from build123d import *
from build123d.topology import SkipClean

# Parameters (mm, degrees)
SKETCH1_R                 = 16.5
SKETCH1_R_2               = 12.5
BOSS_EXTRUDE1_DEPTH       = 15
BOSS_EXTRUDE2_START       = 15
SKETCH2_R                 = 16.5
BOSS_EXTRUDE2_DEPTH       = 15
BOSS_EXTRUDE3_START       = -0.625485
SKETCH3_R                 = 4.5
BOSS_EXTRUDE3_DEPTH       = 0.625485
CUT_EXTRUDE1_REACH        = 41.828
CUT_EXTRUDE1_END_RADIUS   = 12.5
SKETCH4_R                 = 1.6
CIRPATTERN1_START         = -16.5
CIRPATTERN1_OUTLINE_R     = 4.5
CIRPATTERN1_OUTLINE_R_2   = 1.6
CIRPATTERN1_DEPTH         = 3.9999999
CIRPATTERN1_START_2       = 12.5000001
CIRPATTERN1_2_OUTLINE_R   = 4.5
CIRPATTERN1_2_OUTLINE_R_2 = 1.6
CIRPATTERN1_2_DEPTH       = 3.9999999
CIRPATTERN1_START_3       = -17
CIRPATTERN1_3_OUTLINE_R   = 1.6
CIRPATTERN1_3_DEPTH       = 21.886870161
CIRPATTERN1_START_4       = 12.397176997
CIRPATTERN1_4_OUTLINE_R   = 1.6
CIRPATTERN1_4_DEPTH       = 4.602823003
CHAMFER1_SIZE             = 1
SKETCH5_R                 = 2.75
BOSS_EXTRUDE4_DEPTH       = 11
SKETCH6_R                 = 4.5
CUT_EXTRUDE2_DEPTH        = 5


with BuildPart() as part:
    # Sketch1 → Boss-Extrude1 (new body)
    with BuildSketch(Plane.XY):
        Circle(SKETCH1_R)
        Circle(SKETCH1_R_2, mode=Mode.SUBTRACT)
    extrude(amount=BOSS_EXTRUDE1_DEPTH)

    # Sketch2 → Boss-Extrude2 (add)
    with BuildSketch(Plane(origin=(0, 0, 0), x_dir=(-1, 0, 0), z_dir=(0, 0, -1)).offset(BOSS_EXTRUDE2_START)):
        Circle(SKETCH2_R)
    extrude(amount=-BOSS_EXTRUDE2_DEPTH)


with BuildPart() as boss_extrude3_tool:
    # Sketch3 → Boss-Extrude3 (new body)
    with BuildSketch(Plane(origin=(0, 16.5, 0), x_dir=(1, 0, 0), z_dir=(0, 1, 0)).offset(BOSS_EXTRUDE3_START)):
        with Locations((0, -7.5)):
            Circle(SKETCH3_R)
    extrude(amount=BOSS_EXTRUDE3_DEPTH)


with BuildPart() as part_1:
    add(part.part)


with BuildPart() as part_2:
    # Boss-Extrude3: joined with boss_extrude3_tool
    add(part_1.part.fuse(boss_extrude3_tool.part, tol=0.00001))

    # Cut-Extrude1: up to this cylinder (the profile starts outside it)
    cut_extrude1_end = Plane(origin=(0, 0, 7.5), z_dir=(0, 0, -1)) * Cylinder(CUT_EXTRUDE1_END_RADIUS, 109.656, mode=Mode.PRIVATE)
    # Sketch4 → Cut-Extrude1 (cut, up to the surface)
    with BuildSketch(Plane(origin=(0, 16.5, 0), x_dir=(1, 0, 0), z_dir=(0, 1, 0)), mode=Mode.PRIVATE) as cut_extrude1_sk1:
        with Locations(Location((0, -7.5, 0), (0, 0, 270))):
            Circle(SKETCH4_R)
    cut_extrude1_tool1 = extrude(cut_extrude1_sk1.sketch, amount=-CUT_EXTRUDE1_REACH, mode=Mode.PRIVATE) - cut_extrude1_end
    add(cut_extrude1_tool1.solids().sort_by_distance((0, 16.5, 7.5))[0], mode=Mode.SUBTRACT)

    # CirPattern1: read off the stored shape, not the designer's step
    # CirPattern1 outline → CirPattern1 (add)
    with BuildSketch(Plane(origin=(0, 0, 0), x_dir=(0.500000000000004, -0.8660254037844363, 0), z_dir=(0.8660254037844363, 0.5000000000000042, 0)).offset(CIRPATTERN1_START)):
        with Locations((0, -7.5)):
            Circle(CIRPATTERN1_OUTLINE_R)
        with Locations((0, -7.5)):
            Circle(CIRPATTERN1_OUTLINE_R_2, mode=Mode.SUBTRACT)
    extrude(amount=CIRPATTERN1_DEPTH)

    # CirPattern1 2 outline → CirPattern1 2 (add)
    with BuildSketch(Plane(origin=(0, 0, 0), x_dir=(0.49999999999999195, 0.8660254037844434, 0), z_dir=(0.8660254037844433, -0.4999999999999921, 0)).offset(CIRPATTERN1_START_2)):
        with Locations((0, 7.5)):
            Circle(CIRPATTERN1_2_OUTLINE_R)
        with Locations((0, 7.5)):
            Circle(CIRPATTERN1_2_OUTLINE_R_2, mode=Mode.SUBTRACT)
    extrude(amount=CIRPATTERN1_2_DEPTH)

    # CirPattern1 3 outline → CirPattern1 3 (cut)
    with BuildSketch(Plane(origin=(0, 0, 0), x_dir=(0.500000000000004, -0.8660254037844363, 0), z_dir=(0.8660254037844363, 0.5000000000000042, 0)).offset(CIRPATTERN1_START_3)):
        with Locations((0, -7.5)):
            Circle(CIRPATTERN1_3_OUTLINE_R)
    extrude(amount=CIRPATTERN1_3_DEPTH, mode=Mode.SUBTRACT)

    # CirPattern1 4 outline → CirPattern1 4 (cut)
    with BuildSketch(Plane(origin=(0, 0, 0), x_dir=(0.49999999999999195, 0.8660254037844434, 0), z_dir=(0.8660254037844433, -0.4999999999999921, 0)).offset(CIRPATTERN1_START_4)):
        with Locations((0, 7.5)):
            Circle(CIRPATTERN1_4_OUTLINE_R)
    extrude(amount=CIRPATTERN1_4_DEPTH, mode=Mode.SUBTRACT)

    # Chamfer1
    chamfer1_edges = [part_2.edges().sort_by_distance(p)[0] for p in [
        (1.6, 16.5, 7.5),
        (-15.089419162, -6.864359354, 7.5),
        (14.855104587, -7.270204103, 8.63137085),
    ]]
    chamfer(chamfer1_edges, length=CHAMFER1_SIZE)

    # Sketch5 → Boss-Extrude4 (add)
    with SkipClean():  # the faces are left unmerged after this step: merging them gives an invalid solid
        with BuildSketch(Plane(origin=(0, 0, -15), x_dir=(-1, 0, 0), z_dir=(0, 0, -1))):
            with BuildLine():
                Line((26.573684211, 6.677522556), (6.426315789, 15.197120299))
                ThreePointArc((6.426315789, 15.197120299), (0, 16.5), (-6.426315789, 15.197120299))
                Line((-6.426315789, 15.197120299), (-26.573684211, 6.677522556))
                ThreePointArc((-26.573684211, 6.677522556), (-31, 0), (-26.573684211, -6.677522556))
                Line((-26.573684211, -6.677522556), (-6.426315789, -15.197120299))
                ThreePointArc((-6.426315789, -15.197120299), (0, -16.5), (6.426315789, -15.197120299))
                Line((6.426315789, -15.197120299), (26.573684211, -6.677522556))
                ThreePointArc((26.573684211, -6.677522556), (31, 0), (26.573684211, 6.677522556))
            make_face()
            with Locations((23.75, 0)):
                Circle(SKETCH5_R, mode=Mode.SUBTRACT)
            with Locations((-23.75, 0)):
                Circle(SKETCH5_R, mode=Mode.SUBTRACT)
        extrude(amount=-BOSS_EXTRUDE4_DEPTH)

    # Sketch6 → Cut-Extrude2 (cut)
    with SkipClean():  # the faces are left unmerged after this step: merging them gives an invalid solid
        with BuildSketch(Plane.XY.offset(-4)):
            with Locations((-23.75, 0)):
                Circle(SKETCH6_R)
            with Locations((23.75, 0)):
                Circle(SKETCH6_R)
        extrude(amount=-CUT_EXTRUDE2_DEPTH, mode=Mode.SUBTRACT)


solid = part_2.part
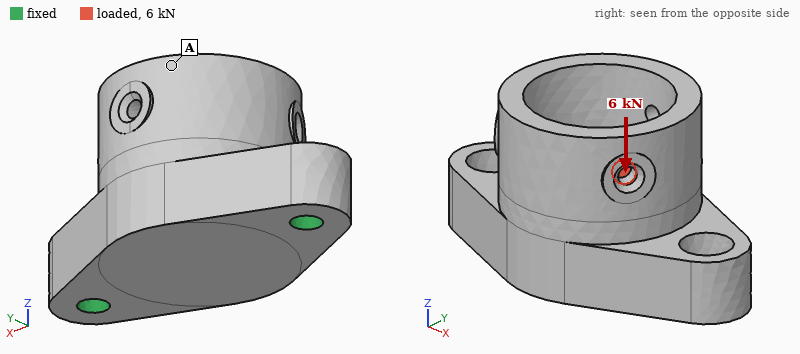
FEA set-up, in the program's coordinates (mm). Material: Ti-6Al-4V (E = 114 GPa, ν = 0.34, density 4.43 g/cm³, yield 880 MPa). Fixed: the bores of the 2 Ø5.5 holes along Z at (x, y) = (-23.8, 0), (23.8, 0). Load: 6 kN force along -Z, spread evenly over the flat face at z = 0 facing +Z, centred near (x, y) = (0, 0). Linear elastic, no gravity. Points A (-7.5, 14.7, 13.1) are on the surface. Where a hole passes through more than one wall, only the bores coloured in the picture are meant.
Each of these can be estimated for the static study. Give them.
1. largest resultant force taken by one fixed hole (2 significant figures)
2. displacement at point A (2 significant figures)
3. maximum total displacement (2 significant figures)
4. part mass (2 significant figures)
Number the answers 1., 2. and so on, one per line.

1. 3.6 kN
2. 12 µm
3. 14 µm
4. 100 g
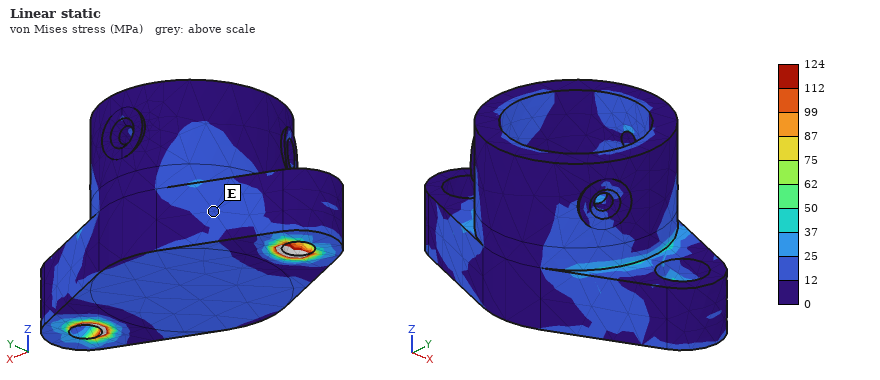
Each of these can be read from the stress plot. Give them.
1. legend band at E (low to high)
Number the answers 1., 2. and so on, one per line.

1. 12 to 25 MPa
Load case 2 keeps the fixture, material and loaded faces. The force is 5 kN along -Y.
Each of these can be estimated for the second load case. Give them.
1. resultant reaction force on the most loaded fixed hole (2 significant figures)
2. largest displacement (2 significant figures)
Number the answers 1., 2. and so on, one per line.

1. 2.5 kN
2. 82 µm
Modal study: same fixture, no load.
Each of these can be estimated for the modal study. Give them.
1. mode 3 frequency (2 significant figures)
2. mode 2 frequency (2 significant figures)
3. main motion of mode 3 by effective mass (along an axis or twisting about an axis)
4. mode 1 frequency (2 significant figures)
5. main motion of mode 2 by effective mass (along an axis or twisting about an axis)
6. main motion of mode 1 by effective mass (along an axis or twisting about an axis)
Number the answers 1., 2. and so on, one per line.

1. 18 kHz
2. 13 kHz
3. along X
4. 5500 Hz
5. along Z
6. along Y
